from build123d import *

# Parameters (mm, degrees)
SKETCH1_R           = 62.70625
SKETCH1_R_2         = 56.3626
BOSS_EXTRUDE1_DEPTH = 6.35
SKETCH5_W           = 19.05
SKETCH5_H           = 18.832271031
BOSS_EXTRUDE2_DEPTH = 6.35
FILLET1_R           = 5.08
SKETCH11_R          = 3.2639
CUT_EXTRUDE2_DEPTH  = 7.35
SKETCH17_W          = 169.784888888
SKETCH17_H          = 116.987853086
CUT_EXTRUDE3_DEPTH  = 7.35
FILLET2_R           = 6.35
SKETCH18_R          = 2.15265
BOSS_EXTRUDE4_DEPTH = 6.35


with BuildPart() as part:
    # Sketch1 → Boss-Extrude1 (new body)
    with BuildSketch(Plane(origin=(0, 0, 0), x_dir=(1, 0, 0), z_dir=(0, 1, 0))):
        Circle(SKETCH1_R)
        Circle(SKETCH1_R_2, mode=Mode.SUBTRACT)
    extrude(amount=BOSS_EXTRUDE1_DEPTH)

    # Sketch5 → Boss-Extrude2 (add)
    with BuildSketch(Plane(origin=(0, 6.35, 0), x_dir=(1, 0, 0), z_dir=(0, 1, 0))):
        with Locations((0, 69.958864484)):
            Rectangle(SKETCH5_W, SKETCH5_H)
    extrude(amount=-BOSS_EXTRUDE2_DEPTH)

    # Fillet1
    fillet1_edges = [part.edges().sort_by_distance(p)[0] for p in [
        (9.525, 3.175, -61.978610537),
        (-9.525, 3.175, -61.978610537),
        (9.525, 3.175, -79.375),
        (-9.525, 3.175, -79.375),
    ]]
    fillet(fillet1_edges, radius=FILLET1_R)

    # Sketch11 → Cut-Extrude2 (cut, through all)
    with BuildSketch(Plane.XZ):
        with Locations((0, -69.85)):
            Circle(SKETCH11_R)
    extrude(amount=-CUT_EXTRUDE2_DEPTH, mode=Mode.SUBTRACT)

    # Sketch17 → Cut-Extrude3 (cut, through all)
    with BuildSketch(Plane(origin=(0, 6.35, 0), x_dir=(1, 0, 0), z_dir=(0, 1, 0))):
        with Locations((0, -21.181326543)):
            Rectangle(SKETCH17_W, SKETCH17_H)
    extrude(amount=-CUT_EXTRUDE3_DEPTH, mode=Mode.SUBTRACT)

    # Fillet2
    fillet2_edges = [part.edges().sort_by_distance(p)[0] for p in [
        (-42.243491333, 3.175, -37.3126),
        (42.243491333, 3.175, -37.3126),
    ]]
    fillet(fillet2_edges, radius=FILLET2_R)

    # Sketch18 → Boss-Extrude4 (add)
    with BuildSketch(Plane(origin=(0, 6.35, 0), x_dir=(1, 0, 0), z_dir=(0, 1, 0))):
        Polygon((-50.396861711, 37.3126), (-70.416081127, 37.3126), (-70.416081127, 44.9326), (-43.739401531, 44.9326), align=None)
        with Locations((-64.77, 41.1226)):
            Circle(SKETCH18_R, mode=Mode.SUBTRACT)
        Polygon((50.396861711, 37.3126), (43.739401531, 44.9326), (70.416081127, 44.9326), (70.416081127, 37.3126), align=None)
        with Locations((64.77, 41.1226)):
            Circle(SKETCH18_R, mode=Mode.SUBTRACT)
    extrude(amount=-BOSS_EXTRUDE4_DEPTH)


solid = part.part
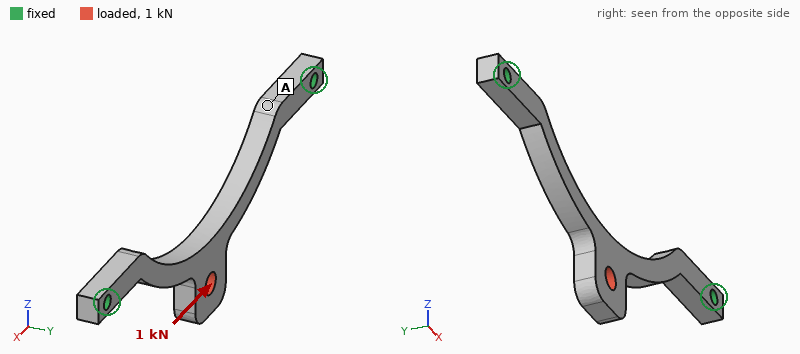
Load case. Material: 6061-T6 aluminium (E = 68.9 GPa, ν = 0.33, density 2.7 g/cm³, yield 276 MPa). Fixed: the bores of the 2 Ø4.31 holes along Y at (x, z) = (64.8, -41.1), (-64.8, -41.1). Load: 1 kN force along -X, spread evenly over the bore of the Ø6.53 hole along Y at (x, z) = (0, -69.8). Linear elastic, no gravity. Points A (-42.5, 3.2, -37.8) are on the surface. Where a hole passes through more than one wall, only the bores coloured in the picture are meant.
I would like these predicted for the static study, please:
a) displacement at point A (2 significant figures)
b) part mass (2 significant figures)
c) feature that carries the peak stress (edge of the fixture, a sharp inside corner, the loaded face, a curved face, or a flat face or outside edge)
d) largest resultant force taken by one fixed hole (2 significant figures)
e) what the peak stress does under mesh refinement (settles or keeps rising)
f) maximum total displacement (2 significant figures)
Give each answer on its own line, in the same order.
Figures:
40 µm
22 g
edge of the fixture
580 N
keeps rising
82 µm
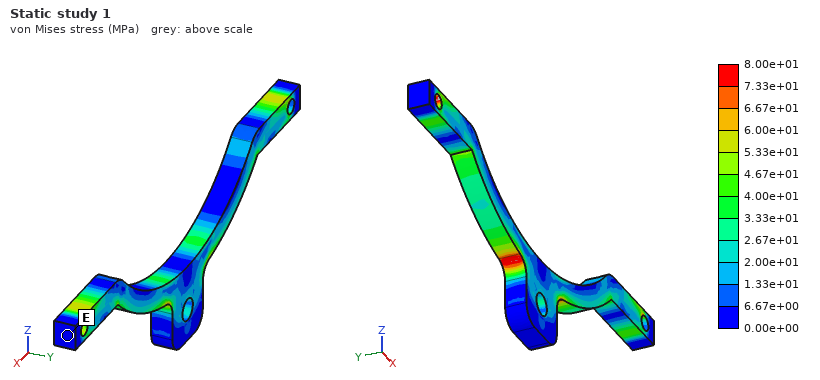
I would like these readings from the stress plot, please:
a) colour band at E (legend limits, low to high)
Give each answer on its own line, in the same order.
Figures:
0.00e+00 to 6.67e+00 MPa
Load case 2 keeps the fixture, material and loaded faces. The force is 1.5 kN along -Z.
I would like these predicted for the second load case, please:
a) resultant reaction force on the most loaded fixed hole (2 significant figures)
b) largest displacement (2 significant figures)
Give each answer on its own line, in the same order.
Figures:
1.7 kN
0.16 mm
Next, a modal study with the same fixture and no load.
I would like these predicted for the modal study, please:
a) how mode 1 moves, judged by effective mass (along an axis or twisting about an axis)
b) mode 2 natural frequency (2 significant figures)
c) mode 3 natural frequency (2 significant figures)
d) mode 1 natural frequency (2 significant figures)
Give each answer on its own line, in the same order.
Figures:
along Y
4100 Hz
4200 Hz
1000 Hz
